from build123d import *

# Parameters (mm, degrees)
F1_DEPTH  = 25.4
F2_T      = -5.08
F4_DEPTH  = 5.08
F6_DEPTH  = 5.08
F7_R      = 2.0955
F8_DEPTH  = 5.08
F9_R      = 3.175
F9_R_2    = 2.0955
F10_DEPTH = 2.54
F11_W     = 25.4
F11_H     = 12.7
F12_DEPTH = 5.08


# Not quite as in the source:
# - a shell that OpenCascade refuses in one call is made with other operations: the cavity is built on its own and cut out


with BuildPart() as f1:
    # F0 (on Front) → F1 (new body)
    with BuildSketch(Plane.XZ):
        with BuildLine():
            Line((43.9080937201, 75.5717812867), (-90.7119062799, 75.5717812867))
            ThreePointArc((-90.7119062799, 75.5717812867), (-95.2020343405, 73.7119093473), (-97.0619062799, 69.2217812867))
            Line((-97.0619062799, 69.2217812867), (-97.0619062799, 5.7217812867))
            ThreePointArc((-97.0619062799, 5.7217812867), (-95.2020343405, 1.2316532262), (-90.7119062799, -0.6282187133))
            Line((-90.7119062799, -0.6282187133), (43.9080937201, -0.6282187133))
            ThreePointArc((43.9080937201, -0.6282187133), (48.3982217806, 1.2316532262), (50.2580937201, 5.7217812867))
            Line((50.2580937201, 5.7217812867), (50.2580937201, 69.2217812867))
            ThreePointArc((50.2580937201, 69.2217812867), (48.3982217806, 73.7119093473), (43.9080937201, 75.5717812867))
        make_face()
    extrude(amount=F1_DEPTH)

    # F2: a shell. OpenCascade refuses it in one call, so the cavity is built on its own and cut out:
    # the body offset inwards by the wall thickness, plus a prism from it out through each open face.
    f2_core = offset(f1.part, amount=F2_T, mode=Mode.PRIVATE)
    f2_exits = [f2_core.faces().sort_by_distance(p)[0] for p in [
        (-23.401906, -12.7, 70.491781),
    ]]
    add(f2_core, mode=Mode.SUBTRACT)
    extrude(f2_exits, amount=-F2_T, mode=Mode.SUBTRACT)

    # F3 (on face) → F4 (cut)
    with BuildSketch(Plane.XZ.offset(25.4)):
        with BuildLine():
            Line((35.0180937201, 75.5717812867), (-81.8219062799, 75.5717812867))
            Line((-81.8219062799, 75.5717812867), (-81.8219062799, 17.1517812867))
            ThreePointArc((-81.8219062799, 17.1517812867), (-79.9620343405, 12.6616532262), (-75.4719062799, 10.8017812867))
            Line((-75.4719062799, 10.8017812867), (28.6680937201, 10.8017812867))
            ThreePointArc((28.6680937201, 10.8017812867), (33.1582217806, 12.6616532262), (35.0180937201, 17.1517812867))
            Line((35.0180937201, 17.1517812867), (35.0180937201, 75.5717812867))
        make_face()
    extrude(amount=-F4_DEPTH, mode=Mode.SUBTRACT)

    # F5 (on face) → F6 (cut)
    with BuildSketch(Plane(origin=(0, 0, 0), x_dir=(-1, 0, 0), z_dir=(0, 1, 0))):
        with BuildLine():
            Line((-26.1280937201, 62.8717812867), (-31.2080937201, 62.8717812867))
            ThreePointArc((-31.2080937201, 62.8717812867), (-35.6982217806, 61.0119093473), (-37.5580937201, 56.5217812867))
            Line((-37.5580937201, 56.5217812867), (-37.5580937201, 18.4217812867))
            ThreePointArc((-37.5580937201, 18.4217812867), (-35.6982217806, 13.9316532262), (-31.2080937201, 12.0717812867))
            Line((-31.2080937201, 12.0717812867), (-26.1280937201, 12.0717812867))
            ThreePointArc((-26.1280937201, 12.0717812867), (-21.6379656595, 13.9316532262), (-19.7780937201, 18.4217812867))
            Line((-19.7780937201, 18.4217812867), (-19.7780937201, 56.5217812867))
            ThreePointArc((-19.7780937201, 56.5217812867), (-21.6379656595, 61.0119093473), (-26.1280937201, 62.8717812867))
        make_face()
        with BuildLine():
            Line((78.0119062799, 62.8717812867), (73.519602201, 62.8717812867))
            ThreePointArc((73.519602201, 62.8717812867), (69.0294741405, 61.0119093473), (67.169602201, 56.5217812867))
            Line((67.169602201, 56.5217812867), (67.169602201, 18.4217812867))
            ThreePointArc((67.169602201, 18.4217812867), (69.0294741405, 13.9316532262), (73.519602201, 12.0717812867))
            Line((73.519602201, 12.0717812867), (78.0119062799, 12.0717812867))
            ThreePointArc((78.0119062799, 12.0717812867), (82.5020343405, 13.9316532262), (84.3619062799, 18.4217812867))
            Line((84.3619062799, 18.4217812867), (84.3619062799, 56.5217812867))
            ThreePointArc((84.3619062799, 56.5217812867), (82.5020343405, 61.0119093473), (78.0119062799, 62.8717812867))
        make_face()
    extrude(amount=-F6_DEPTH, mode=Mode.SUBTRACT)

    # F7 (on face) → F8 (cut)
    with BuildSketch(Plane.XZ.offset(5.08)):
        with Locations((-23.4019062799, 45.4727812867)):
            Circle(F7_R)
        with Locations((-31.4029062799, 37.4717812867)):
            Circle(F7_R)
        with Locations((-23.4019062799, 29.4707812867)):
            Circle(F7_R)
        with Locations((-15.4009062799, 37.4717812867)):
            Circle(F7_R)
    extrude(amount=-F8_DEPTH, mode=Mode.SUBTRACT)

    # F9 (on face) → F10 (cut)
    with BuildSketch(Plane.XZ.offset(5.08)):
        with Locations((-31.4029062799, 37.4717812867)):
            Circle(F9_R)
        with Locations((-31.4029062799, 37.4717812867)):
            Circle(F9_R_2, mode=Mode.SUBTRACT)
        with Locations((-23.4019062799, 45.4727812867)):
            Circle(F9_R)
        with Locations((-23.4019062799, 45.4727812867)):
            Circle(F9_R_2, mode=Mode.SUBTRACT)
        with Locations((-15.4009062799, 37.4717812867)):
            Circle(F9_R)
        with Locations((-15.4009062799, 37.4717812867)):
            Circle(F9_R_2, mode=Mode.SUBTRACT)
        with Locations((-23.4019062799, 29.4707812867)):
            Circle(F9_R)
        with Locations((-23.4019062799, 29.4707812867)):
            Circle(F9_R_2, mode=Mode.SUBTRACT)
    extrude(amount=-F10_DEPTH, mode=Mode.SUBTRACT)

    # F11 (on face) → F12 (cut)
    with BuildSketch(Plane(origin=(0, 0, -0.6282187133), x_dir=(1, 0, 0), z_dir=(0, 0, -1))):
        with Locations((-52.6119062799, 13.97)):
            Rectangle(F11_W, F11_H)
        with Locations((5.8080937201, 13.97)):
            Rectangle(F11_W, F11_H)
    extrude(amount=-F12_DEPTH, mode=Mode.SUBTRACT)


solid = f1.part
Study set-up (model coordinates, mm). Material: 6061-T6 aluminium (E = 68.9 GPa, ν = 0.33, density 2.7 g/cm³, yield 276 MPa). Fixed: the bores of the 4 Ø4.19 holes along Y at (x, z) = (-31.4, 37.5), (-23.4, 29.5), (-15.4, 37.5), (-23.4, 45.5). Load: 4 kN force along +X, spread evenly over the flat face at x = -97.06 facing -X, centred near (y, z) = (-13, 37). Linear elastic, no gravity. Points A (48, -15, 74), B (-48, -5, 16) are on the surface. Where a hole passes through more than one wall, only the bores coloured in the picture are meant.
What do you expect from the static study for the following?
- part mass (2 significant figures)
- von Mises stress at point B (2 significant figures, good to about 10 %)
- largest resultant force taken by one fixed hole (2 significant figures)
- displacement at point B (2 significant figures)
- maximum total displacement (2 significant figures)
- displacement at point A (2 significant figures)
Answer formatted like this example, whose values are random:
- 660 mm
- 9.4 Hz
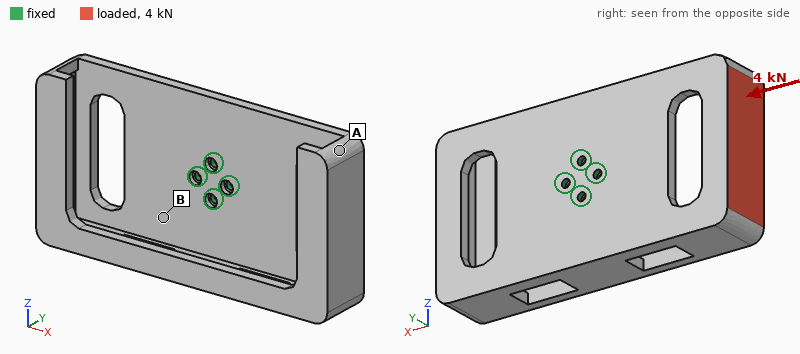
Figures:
- 230 g
- 40 MPa
- 2.2 kN
- 0.20 mm
- 0.92 mm
- 0.39 mm
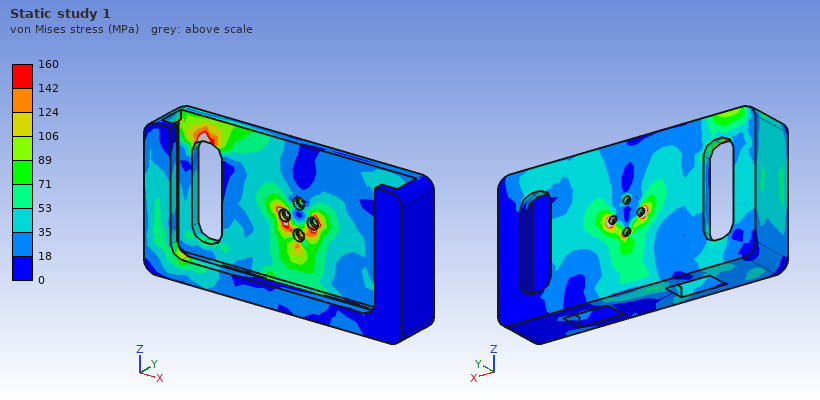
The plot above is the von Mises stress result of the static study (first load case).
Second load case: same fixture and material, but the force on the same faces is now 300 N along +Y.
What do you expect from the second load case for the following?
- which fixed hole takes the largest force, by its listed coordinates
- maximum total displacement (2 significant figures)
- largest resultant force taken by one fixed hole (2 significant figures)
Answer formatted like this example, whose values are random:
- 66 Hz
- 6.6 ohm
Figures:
- (-31.4, 37.5)
- 0.42 mm
- 1.2 kN
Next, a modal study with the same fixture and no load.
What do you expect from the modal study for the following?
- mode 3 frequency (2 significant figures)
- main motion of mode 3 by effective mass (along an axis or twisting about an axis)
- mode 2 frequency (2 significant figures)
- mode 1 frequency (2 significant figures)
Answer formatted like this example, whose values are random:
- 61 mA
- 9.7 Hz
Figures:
- 1000 Hz
- along Y
- 830 Hz
- 480 Hz
